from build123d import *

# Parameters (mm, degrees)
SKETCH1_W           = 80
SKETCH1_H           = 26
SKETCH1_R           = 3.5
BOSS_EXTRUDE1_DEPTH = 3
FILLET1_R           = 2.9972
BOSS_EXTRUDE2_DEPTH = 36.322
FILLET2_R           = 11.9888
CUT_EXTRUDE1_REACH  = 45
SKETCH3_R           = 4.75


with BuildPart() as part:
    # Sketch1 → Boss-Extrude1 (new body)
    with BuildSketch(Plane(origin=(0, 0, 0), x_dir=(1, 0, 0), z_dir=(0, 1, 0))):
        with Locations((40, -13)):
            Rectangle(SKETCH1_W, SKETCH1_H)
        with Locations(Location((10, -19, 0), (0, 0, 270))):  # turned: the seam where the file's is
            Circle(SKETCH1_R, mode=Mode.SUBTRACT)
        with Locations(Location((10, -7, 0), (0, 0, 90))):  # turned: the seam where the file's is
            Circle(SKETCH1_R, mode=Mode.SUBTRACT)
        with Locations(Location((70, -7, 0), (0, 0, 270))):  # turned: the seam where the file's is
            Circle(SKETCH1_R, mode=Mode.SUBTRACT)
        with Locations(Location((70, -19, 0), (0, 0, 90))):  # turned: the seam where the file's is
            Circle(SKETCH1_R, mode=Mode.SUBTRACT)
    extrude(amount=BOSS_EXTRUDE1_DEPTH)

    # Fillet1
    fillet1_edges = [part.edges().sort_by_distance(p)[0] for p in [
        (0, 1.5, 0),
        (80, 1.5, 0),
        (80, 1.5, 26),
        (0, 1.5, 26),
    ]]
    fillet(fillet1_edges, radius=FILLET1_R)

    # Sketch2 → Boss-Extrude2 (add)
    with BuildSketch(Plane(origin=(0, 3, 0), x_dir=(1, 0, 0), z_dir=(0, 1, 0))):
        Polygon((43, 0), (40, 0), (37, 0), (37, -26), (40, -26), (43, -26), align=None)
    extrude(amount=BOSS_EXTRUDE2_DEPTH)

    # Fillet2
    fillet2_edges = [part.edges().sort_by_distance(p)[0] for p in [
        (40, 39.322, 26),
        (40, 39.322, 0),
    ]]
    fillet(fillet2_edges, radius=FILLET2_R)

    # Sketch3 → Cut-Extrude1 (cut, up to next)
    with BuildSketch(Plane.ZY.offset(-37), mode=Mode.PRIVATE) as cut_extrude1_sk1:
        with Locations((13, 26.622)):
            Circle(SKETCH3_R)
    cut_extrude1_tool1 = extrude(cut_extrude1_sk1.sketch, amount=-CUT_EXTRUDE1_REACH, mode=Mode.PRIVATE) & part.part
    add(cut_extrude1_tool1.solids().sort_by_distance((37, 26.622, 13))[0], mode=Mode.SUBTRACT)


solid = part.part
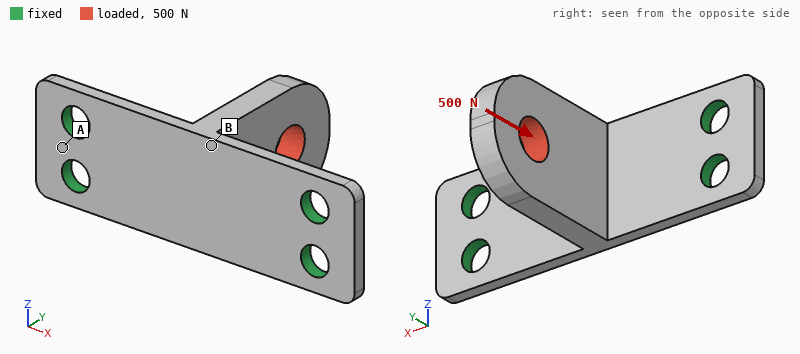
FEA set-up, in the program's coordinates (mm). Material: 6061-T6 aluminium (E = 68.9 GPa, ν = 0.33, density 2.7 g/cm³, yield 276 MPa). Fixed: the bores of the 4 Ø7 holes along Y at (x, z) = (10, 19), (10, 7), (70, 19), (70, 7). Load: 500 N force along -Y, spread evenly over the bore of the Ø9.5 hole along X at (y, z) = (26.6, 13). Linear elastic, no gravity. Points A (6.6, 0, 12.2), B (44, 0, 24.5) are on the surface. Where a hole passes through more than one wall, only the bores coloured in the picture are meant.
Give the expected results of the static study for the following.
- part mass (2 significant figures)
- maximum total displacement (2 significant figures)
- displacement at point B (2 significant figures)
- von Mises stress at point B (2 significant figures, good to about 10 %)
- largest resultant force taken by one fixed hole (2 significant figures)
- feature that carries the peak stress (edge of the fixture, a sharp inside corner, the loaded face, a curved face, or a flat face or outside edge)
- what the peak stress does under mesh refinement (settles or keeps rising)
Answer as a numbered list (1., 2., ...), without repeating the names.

1. 29 g
2. 87 µm
3. 83 µm
4. 56 MPa
5. 130 N
6. edge of the fixture
7. keeps rising
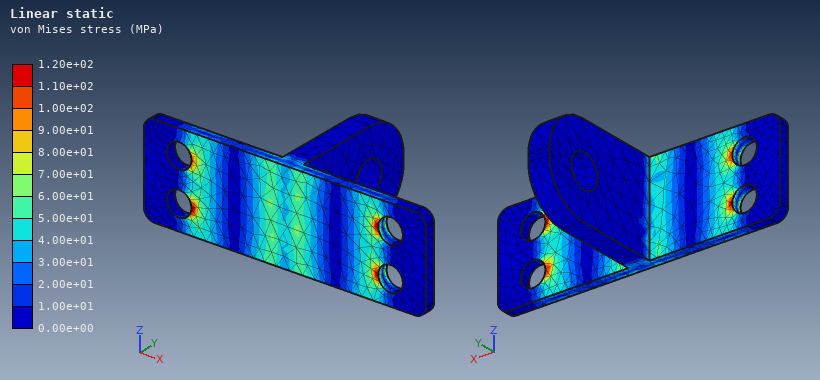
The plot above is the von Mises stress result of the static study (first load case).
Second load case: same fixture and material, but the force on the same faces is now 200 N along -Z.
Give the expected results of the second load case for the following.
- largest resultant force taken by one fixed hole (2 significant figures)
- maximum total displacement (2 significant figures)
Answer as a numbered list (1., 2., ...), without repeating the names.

1. 180 N
2. 0.25 mm
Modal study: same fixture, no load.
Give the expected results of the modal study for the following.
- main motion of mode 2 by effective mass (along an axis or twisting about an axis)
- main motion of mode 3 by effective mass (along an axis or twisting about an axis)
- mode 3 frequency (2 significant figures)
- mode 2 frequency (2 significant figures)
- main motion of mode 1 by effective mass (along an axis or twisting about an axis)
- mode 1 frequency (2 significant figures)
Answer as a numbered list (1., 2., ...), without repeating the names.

1. along X
2. along Y
3. 2900 Hz
4. 2300 Hz
5. along Z
6. 1700 Hz
